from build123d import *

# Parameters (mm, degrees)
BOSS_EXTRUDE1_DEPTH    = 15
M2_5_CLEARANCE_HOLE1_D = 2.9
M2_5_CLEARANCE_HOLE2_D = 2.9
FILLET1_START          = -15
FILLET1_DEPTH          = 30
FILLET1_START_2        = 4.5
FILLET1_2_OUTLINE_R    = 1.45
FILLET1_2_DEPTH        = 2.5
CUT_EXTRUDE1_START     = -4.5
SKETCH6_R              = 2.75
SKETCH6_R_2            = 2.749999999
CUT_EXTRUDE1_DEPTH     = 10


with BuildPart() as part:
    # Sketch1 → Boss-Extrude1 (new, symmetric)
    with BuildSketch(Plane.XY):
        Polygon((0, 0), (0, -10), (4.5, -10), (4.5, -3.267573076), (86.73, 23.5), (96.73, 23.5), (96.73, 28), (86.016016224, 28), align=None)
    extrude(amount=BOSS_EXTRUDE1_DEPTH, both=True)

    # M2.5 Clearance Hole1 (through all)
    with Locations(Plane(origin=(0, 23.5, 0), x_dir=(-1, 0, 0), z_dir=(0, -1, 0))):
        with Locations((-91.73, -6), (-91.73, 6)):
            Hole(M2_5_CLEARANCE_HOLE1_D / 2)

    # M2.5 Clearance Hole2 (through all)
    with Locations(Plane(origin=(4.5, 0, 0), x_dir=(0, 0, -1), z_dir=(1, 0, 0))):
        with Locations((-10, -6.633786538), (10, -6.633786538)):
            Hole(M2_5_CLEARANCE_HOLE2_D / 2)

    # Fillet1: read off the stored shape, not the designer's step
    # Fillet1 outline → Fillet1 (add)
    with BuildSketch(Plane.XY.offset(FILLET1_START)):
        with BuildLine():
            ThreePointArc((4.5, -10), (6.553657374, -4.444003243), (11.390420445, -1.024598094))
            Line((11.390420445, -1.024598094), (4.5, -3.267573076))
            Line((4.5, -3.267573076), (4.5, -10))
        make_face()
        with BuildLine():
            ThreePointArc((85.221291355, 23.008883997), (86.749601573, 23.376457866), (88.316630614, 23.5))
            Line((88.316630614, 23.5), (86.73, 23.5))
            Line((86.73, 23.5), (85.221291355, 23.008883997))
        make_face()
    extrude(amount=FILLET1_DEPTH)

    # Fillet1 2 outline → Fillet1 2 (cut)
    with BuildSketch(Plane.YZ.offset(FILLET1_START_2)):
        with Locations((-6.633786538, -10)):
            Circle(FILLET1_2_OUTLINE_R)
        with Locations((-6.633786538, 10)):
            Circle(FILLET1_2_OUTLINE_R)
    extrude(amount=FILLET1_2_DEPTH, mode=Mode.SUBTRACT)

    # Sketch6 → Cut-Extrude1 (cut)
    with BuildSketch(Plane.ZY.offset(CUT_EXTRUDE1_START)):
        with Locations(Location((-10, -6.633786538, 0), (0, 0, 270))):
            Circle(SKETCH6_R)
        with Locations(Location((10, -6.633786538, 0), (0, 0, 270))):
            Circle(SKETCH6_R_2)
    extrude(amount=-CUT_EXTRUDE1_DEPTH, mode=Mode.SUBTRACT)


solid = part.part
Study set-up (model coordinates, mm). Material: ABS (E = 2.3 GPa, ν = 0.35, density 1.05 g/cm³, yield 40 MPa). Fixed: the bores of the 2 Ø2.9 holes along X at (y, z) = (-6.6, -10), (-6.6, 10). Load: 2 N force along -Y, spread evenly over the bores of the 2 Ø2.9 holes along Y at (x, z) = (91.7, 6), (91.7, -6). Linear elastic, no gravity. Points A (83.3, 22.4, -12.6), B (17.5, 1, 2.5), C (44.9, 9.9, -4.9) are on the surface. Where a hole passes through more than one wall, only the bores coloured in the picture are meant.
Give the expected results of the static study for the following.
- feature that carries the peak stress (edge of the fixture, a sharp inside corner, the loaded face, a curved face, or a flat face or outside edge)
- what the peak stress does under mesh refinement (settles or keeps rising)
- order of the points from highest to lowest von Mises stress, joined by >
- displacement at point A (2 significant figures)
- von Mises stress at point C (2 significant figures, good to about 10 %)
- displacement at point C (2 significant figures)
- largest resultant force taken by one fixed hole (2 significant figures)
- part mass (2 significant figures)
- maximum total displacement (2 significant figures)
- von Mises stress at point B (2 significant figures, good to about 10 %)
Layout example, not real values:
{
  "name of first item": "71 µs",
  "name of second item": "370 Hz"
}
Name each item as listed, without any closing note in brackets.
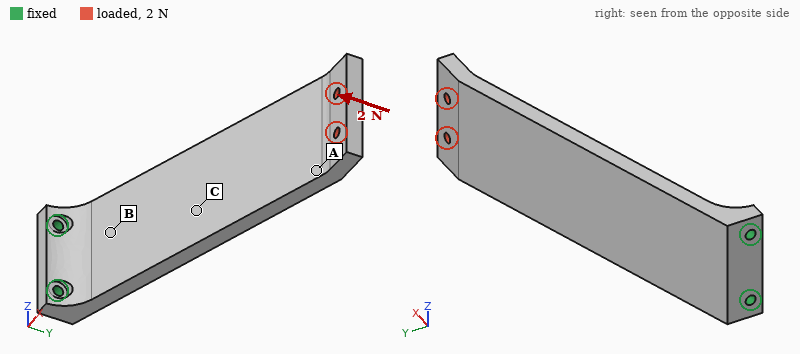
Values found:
{
  "feature that carries the peak stress": "edge of the fixture",
  "what the peak stress does under mesh refinement": "keeps rising",
  "order of the points from highest to lowest von Mises stress, joined by >": "B > C > A",
  "displacement at point A": "0.87 mm",
  "von Mises stress at point C": "0.94 MPa",
  "displacement at point C": "0.29 mm",
  "largest resultant force taken by one fixed hole": "3.0 N",
  "part mass": "15 g",
  "maximum total displacement": "1.1 mm",
  "von Mises stress at point B": "1.4 MPa"
}
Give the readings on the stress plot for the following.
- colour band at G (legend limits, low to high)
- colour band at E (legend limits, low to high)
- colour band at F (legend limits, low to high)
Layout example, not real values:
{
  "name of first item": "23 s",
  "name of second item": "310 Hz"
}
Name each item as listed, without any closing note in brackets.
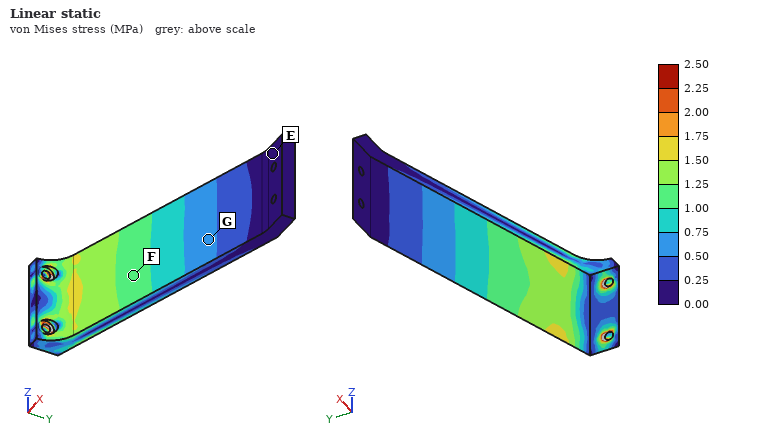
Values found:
{
  "colour band at G": "0.50 to 0.75 MPa",
  "colour band at E": "0.00 to 0.25 MPa",
  "colour band at F": "1.00 to 1.25 MPa"
}
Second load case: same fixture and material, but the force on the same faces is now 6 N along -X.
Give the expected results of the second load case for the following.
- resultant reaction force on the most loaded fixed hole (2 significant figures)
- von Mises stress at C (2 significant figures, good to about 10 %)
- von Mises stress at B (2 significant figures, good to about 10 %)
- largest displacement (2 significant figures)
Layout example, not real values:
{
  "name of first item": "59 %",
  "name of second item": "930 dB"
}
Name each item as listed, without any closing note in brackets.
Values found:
{
  "resultant reaction force on the most loaded fixed hole": "3.7 N",
  "von Mises stress at C": "0.76 MPa",
  "von Mises stress at B": "1.3 MPa",
  "largest displacement": "1.00 mm"
}
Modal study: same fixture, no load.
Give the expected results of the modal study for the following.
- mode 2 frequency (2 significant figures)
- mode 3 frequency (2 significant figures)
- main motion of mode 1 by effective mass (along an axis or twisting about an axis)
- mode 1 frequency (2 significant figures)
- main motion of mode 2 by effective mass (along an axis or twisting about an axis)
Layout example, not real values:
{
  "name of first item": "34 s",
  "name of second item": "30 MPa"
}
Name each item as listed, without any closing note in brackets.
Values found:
{
  "mode 2 frequency": "540 Hz",
  "mode 3 frequency": "670 Hz",
  "main motion of mode 1 by effective mass": "along Y",
  "mode 1 frequency": "110 Hz",
  "main motion of mode 2 by effective mass": "along Z"
}
